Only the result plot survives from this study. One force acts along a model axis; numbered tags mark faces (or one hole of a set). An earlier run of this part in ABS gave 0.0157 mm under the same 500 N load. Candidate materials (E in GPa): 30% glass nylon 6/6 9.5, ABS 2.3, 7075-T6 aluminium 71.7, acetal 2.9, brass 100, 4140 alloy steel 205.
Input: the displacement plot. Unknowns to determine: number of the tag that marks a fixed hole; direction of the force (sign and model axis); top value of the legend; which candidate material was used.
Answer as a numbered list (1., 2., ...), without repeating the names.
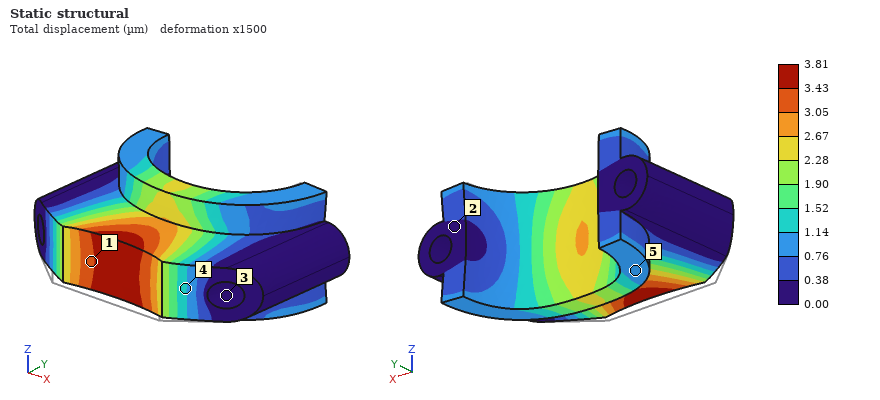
1. 3
2. +Y
3. 3.81 µm
4. 30% glass nylon 6/6
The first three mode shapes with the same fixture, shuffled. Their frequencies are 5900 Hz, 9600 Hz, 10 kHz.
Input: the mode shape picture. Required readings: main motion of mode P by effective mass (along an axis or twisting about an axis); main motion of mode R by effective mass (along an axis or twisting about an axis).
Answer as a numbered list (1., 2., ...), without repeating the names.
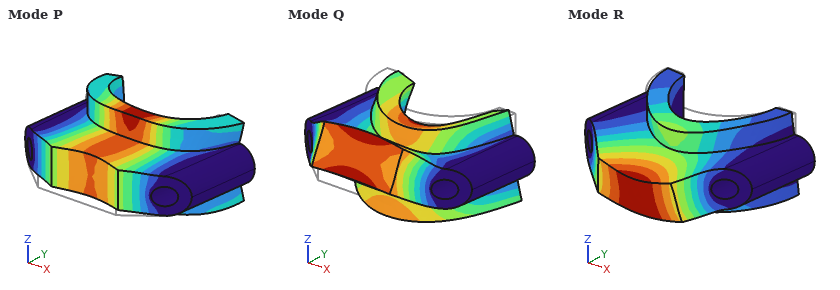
1. along Y
2. along Z
